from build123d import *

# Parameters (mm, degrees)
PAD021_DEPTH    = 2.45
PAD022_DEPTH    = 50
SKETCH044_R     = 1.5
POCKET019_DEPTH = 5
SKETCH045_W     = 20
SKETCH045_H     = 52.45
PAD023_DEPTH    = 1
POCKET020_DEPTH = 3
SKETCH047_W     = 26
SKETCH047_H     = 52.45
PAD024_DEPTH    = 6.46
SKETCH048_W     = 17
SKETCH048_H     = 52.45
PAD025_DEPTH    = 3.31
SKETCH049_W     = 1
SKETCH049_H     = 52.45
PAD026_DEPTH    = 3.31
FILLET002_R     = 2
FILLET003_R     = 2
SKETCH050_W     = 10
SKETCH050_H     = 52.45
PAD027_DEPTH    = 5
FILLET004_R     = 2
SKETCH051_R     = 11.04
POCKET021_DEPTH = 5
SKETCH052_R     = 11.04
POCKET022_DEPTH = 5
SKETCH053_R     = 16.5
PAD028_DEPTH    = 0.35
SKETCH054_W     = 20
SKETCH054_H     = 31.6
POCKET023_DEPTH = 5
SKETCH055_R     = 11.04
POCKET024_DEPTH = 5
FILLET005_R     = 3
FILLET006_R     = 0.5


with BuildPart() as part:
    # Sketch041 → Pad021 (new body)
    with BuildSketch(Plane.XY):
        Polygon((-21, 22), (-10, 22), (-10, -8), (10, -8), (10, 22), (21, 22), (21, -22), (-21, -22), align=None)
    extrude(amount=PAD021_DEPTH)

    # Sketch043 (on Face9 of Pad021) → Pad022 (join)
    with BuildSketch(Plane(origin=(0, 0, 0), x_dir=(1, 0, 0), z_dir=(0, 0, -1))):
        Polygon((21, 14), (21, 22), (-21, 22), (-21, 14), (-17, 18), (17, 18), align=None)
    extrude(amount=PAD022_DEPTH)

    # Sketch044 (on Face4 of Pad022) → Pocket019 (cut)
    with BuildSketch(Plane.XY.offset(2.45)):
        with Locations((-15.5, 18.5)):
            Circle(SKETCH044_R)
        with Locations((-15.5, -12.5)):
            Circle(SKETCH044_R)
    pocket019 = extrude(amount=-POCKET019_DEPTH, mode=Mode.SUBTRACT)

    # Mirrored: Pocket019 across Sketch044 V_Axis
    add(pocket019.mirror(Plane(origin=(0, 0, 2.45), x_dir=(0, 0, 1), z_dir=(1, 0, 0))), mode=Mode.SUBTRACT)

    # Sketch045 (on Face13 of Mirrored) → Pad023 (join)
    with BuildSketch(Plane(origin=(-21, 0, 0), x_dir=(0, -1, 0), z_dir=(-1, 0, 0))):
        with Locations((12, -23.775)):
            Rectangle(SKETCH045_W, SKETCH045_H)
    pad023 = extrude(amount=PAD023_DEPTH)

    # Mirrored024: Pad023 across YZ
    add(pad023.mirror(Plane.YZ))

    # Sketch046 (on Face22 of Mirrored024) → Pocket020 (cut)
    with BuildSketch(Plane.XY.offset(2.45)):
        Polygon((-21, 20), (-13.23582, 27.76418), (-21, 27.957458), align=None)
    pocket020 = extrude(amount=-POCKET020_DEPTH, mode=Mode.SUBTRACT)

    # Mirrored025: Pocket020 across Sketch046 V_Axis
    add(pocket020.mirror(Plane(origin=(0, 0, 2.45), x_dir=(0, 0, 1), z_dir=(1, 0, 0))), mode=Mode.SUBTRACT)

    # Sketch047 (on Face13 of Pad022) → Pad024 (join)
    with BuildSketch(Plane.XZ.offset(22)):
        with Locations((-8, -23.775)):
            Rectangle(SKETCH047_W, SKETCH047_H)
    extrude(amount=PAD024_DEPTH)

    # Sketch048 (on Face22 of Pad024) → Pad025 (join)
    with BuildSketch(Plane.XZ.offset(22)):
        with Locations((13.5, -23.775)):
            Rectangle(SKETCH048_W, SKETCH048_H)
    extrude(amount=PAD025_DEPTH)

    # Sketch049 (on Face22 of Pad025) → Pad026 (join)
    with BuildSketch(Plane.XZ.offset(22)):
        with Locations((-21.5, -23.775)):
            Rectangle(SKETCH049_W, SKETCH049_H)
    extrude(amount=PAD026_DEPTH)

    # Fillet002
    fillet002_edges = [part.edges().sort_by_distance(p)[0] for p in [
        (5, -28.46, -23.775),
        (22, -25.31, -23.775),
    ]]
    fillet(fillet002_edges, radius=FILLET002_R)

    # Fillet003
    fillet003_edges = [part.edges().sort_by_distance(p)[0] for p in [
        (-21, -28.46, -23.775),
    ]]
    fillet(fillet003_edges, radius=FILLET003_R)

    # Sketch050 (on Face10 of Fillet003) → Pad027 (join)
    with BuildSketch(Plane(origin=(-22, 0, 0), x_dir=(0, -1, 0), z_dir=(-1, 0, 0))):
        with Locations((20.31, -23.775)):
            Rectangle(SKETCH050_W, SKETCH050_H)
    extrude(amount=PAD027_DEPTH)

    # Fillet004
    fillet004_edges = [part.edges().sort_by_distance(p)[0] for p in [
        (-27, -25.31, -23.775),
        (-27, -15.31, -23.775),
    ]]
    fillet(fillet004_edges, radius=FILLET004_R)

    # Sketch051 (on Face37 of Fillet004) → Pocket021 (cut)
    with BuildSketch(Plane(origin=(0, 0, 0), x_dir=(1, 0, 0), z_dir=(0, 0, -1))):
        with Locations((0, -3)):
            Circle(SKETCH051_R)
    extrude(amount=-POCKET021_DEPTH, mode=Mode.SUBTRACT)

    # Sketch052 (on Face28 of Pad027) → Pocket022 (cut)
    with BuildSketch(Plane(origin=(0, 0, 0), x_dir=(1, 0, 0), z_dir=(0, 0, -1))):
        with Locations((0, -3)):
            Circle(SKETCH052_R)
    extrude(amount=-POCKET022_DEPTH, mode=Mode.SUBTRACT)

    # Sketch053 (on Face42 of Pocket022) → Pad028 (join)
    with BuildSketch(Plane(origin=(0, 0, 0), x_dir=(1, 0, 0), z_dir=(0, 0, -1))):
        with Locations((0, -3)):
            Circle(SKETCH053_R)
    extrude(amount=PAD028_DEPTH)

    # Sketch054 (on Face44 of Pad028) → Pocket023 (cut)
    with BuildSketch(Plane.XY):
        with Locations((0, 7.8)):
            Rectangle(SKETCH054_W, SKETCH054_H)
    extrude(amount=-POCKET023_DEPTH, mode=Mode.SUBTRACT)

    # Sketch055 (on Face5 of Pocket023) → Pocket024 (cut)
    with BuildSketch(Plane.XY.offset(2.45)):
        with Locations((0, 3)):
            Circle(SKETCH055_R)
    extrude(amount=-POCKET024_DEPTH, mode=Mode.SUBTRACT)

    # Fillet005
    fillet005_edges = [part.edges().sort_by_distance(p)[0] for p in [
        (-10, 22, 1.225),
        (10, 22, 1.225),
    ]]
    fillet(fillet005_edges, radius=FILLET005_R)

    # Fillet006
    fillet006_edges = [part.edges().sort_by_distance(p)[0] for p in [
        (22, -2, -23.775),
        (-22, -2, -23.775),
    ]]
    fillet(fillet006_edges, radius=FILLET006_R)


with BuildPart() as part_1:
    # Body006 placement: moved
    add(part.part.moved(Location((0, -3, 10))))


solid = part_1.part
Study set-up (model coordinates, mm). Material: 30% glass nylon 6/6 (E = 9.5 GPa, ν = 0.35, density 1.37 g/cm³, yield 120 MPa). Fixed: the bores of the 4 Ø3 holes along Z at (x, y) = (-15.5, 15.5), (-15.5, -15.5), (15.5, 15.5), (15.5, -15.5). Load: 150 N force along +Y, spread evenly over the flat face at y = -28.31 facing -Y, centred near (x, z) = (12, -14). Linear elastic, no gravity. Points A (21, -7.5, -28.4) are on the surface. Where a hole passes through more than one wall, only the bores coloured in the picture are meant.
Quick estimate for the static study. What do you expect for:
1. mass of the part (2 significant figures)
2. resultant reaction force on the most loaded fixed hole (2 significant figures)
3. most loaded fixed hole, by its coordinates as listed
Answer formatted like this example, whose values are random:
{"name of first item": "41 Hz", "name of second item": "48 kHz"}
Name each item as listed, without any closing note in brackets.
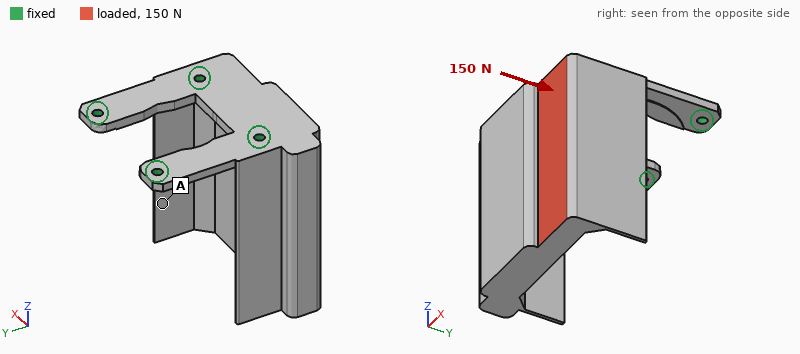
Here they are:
{"mass of the part": "39 g", "resultant reaction force on the most loaded fixed hole": "110 N", "most loaded fixed hole, by its coordinates as listed": "(15.5, -15.5)"}
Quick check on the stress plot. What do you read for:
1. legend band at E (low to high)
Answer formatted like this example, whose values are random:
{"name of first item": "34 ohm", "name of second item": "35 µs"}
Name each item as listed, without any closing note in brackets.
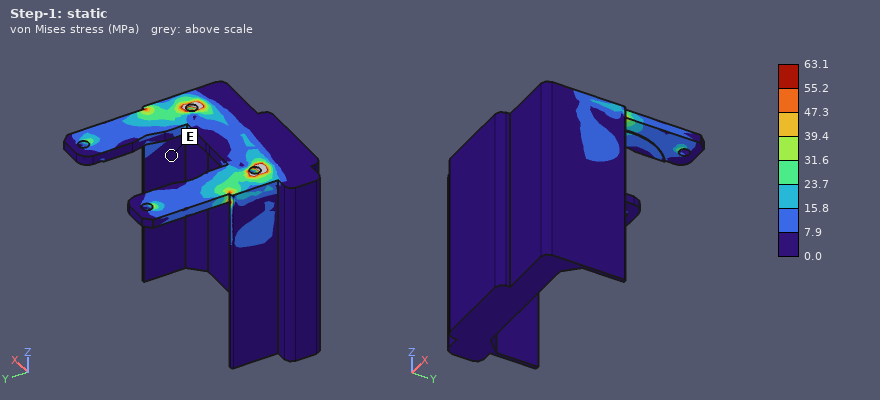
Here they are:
{"legend band at E": "0.0 to 7.9 MPa"}
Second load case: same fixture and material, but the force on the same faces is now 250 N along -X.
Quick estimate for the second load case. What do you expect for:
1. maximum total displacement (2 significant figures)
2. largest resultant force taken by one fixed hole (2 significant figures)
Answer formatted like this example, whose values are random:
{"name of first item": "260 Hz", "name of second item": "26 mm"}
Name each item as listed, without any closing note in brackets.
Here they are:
{"maximum total displacement": "0.12 mm", "largest resultant force taken by one fixed hole": "240 N"}
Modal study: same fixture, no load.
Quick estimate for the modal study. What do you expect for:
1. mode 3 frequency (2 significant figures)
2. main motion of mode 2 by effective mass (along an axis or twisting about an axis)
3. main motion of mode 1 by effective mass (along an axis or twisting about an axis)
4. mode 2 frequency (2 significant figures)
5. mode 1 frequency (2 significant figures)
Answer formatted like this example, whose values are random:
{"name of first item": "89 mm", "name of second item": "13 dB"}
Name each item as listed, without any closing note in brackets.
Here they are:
{"mode 3 frequency": "2600 Hz", "main motion of mode 2 by effective mass": "along X", "main motion of mode 1 by effective mass": "along Y", "mode 2 frequency": "1400 Hz", "mode 1 frequency": "400 Hz"}
